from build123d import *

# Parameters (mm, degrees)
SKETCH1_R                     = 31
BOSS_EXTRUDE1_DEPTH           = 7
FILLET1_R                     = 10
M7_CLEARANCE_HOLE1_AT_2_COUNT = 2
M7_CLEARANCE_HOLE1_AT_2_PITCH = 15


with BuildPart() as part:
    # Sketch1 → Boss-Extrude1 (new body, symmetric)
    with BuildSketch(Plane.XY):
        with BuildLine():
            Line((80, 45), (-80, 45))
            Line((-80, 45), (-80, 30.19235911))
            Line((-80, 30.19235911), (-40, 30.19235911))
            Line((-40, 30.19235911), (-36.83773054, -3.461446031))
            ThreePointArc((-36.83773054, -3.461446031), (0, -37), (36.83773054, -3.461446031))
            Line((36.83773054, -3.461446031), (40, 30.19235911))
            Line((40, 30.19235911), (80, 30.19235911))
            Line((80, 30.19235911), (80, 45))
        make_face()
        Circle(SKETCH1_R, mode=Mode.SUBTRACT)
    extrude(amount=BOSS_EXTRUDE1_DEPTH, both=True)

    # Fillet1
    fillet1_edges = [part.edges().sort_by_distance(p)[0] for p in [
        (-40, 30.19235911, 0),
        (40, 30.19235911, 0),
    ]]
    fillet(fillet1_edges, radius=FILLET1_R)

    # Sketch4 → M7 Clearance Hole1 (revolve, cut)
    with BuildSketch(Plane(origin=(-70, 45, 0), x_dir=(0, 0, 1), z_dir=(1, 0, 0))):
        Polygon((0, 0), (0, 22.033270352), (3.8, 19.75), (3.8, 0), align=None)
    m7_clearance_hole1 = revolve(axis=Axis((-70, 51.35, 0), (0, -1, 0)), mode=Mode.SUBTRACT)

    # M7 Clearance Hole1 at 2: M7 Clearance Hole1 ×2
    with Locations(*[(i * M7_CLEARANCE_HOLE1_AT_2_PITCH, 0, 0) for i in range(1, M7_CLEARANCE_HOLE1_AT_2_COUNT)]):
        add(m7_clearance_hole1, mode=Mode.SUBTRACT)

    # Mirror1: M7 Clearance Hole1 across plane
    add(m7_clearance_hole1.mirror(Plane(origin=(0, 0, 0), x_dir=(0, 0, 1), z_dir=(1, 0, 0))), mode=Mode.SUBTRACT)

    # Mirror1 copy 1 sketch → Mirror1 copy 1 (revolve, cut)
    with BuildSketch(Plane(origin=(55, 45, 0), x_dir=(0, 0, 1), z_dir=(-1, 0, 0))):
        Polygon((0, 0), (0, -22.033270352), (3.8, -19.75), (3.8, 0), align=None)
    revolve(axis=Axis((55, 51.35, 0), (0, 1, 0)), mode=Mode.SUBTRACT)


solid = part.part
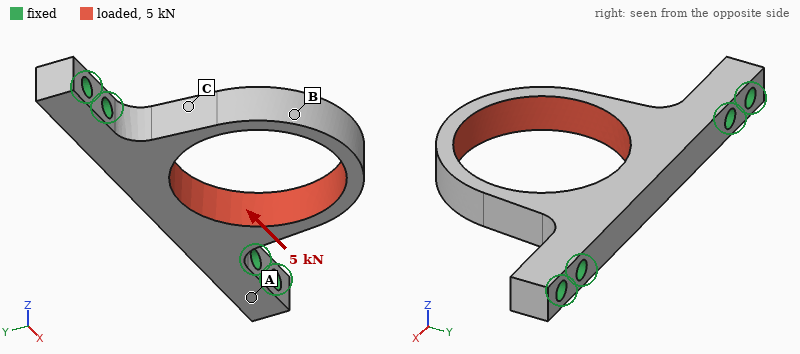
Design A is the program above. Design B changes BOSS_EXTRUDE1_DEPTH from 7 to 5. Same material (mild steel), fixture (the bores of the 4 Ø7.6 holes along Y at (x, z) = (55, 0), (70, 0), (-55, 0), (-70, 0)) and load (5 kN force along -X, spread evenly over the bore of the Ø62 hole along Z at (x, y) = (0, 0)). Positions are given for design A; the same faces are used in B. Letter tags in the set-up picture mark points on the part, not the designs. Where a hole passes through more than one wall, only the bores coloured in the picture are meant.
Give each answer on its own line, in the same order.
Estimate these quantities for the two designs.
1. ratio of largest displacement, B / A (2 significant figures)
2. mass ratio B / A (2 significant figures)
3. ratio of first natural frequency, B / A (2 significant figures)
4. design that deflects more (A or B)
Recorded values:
1.4
0.70
0.78
B
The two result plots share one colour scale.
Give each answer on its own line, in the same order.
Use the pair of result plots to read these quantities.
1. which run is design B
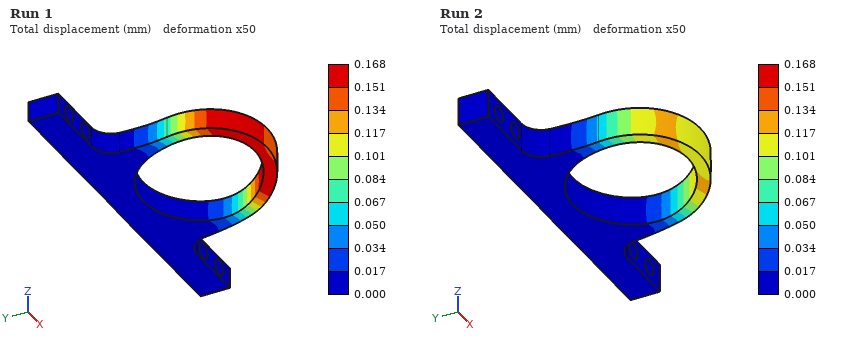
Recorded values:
Run 1
